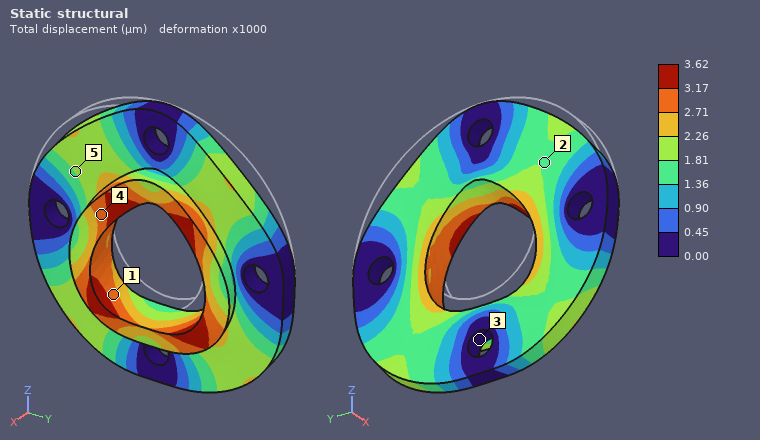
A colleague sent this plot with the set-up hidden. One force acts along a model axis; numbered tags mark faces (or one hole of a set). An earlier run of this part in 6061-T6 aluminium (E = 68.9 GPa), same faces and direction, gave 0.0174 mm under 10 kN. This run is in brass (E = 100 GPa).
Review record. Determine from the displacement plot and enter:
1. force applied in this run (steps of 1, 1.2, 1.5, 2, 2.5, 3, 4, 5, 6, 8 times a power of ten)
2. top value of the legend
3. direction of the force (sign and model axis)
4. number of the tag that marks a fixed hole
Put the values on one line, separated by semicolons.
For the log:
3 kN; 3.62 µm; -Z; 3
